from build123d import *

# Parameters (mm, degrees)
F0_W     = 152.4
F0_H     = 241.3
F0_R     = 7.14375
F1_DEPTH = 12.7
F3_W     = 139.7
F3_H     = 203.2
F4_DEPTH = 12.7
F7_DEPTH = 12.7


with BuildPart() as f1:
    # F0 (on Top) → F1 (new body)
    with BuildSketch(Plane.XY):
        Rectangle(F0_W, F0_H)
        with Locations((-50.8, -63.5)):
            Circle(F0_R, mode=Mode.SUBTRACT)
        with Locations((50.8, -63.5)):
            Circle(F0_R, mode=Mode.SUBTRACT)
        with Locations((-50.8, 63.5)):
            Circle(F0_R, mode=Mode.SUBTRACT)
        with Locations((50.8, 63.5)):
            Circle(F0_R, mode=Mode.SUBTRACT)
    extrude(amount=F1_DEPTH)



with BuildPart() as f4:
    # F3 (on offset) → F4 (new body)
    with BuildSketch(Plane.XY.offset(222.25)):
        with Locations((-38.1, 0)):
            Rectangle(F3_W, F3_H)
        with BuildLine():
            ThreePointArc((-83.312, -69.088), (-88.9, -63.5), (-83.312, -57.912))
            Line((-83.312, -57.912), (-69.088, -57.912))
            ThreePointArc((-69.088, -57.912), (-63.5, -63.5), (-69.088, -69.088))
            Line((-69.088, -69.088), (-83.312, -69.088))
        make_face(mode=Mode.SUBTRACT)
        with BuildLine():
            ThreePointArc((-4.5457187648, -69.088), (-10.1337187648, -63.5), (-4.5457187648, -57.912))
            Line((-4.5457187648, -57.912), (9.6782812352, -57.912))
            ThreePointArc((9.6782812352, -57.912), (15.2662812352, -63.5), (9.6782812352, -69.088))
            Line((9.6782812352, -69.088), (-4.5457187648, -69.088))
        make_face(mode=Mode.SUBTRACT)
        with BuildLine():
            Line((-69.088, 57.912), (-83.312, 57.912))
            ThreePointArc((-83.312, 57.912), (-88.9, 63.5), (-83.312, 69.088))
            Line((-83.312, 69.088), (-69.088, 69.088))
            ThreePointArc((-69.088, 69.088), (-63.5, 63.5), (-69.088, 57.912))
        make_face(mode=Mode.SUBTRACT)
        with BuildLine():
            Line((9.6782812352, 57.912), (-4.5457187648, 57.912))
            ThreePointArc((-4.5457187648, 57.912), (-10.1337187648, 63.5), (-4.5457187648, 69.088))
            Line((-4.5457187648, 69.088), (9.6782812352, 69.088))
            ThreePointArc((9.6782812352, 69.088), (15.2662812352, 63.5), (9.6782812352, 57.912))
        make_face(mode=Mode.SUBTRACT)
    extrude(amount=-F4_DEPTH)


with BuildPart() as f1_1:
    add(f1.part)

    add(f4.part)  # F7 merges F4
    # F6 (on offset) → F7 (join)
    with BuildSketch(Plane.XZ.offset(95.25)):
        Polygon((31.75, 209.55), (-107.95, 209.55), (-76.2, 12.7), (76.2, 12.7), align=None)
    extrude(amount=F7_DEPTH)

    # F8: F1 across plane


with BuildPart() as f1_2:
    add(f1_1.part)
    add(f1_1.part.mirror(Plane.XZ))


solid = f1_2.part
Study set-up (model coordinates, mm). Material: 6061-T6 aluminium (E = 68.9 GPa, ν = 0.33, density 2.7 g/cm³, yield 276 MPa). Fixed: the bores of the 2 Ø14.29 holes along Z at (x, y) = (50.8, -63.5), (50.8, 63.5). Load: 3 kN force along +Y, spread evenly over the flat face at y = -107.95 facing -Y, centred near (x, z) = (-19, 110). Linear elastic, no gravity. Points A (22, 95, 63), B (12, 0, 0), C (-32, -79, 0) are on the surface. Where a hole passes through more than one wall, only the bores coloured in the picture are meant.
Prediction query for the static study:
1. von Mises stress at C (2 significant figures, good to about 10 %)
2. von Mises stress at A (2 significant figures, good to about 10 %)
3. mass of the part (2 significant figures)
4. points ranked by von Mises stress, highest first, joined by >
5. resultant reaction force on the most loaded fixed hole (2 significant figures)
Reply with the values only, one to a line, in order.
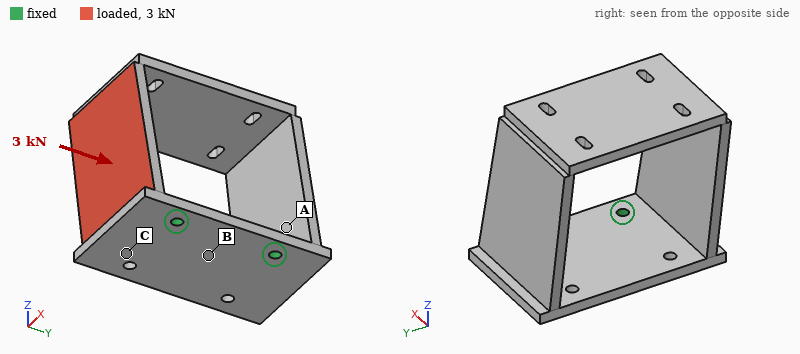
23 MPa
11 MPa
4.1 kg
C > A > B
2.6 kN
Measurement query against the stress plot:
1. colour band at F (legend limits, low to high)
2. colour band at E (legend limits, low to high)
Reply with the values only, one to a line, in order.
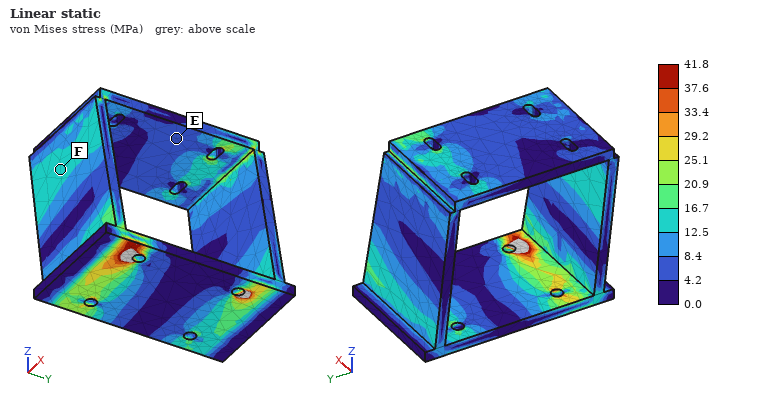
12.5 to 16.7 MPa
4.2 to 8.4 MPa
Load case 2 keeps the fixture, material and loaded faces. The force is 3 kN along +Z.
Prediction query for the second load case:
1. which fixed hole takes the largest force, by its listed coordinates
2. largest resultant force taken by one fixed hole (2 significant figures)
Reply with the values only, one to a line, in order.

(50.8, -63.5)
3.3 kN
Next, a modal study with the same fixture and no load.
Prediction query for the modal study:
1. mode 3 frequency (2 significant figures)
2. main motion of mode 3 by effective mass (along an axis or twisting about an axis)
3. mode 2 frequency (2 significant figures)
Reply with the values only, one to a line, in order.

360 Hz
twisting about Z
170 Hz
